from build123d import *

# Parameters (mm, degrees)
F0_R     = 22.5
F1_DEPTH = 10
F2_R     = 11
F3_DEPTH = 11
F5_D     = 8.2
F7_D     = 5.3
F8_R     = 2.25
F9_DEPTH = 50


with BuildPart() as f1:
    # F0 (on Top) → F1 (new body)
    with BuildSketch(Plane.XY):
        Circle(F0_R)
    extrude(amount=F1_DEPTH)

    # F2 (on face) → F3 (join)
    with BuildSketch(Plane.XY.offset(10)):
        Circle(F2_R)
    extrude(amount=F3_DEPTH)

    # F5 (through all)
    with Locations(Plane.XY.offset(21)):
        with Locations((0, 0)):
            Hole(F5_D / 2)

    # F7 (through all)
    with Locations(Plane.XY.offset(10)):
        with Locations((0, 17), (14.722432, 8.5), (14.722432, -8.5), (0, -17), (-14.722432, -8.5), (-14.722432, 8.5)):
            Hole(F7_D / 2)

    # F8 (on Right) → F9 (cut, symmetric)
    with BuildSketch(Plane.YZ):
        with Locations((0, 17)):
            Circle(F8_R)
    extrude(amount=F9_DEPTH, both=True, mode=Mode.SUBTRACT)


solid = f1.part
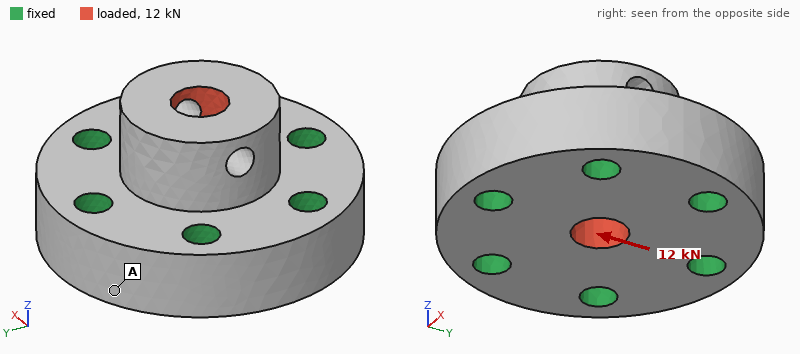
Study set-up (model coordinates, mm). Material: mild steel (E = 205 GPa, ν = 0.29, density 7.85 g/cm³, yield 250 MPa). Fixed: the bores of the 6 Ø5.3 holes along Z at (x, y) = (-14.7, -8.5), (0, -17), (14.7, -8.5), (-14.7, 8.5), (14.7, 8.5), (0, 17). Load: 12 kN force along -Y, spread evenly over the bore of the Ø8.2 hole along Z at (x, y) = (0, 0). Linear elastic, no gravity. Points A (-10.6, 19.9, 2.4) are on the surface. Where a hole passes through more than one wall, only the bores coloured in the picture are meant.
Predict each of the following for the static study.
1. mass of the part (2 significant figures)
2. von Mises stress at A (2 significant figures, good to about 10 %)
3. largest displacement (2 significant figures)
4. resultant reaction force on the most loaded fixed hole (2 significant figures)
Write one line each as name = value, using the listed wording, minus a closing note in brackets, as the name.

mass of the part = 140 g
von Mises stress at A = 8.7 MPa
largest displacement = 6.1 µm
resultant reaction force on the most loaded fixed hole = 3.4 kN
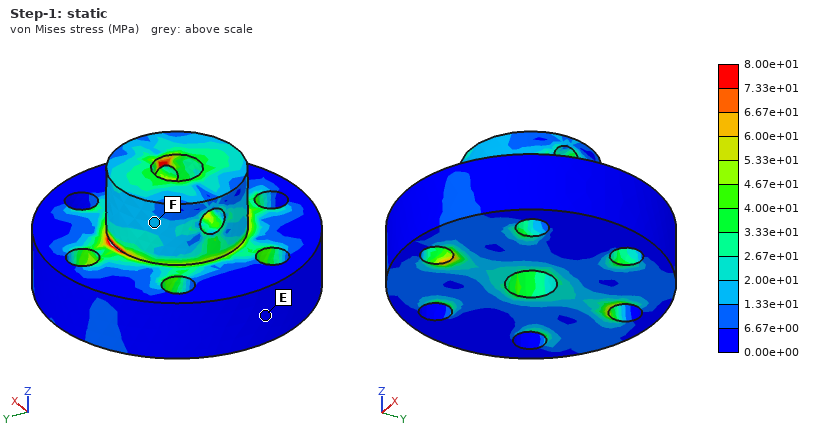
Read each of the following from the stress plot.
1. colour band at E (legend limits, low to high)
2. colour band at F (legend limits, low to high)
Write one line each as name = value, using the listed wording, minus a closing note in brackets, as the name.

colour band at E = 0.00e+00 to 6.67e+00 MPa
colour band at F = 1.33e+01 to 2.00e+01 MPa
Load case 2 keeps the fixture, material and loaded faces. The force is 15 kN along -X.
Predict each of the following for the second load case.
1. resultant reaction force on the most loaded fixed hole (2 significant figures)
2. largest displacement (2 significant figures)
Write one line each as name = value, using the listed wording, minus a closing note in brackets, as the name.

resultant reaction force on the most loaded fixed hole = 3.7 kN
largest displacement = 6.8 µm
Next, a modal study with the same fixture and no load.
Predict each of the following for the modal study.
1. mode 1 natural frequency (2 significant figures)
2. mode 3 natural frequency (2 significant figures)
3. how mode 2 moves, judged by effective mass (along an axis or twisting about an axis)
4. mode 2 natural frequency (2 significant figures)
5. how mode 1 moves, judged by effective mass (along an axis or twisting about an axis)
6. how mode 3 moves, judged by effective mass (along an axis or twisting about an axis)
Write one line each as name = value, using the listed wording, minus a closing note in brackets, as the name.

mode 1 natural frequency = 38 kHz
mode 3 natural frequency = 47 kHz
how mode 2 moves, judged by effective mass = along X
mode 2 natural frequency = 40 kHz
how mode 1 moves, judged by effective mass = along Y
how mode 3 moves, judged by effective mass = along Z
